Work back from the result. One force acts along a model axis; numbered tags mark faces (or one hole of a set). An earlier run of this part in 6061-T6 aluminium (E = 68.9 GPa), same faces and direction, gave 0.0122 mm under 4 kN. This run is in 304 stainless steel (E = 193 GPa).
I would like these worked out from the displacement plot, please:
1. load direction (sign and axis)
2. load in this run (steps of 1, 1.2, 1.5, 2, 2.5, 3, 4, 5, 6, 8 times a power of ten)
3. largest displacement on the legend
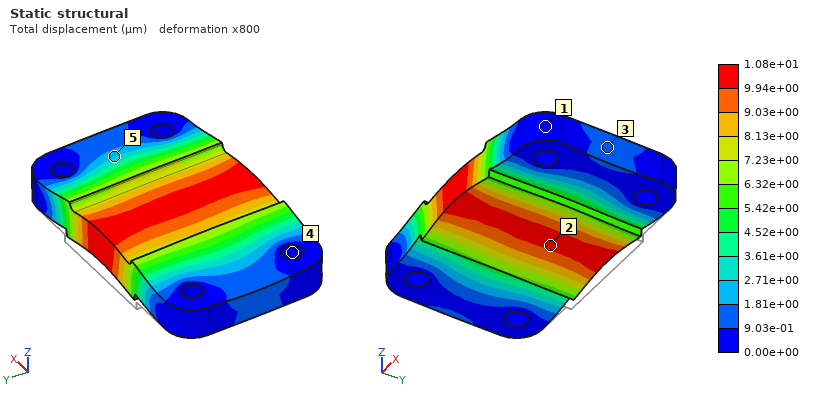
+Z
10 kN
1.08e+01 µm
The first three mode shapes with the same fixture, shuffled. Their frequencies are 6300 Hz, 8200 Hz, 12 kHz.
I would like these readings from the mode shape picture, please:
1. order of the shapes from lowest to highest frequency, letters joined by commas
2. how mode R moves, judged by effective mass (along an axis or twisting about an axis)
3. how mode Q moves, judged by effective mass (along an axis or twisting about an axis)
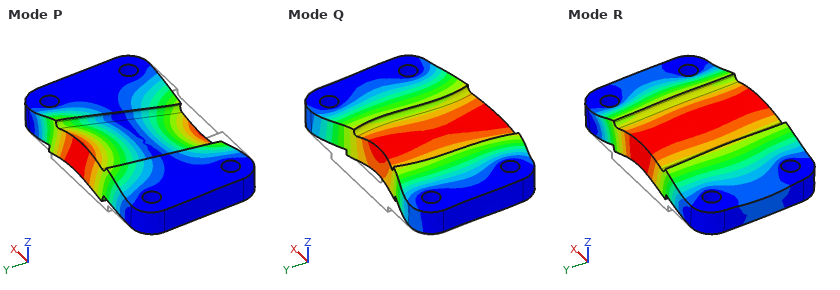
R, P, Q
along Z
along Y
